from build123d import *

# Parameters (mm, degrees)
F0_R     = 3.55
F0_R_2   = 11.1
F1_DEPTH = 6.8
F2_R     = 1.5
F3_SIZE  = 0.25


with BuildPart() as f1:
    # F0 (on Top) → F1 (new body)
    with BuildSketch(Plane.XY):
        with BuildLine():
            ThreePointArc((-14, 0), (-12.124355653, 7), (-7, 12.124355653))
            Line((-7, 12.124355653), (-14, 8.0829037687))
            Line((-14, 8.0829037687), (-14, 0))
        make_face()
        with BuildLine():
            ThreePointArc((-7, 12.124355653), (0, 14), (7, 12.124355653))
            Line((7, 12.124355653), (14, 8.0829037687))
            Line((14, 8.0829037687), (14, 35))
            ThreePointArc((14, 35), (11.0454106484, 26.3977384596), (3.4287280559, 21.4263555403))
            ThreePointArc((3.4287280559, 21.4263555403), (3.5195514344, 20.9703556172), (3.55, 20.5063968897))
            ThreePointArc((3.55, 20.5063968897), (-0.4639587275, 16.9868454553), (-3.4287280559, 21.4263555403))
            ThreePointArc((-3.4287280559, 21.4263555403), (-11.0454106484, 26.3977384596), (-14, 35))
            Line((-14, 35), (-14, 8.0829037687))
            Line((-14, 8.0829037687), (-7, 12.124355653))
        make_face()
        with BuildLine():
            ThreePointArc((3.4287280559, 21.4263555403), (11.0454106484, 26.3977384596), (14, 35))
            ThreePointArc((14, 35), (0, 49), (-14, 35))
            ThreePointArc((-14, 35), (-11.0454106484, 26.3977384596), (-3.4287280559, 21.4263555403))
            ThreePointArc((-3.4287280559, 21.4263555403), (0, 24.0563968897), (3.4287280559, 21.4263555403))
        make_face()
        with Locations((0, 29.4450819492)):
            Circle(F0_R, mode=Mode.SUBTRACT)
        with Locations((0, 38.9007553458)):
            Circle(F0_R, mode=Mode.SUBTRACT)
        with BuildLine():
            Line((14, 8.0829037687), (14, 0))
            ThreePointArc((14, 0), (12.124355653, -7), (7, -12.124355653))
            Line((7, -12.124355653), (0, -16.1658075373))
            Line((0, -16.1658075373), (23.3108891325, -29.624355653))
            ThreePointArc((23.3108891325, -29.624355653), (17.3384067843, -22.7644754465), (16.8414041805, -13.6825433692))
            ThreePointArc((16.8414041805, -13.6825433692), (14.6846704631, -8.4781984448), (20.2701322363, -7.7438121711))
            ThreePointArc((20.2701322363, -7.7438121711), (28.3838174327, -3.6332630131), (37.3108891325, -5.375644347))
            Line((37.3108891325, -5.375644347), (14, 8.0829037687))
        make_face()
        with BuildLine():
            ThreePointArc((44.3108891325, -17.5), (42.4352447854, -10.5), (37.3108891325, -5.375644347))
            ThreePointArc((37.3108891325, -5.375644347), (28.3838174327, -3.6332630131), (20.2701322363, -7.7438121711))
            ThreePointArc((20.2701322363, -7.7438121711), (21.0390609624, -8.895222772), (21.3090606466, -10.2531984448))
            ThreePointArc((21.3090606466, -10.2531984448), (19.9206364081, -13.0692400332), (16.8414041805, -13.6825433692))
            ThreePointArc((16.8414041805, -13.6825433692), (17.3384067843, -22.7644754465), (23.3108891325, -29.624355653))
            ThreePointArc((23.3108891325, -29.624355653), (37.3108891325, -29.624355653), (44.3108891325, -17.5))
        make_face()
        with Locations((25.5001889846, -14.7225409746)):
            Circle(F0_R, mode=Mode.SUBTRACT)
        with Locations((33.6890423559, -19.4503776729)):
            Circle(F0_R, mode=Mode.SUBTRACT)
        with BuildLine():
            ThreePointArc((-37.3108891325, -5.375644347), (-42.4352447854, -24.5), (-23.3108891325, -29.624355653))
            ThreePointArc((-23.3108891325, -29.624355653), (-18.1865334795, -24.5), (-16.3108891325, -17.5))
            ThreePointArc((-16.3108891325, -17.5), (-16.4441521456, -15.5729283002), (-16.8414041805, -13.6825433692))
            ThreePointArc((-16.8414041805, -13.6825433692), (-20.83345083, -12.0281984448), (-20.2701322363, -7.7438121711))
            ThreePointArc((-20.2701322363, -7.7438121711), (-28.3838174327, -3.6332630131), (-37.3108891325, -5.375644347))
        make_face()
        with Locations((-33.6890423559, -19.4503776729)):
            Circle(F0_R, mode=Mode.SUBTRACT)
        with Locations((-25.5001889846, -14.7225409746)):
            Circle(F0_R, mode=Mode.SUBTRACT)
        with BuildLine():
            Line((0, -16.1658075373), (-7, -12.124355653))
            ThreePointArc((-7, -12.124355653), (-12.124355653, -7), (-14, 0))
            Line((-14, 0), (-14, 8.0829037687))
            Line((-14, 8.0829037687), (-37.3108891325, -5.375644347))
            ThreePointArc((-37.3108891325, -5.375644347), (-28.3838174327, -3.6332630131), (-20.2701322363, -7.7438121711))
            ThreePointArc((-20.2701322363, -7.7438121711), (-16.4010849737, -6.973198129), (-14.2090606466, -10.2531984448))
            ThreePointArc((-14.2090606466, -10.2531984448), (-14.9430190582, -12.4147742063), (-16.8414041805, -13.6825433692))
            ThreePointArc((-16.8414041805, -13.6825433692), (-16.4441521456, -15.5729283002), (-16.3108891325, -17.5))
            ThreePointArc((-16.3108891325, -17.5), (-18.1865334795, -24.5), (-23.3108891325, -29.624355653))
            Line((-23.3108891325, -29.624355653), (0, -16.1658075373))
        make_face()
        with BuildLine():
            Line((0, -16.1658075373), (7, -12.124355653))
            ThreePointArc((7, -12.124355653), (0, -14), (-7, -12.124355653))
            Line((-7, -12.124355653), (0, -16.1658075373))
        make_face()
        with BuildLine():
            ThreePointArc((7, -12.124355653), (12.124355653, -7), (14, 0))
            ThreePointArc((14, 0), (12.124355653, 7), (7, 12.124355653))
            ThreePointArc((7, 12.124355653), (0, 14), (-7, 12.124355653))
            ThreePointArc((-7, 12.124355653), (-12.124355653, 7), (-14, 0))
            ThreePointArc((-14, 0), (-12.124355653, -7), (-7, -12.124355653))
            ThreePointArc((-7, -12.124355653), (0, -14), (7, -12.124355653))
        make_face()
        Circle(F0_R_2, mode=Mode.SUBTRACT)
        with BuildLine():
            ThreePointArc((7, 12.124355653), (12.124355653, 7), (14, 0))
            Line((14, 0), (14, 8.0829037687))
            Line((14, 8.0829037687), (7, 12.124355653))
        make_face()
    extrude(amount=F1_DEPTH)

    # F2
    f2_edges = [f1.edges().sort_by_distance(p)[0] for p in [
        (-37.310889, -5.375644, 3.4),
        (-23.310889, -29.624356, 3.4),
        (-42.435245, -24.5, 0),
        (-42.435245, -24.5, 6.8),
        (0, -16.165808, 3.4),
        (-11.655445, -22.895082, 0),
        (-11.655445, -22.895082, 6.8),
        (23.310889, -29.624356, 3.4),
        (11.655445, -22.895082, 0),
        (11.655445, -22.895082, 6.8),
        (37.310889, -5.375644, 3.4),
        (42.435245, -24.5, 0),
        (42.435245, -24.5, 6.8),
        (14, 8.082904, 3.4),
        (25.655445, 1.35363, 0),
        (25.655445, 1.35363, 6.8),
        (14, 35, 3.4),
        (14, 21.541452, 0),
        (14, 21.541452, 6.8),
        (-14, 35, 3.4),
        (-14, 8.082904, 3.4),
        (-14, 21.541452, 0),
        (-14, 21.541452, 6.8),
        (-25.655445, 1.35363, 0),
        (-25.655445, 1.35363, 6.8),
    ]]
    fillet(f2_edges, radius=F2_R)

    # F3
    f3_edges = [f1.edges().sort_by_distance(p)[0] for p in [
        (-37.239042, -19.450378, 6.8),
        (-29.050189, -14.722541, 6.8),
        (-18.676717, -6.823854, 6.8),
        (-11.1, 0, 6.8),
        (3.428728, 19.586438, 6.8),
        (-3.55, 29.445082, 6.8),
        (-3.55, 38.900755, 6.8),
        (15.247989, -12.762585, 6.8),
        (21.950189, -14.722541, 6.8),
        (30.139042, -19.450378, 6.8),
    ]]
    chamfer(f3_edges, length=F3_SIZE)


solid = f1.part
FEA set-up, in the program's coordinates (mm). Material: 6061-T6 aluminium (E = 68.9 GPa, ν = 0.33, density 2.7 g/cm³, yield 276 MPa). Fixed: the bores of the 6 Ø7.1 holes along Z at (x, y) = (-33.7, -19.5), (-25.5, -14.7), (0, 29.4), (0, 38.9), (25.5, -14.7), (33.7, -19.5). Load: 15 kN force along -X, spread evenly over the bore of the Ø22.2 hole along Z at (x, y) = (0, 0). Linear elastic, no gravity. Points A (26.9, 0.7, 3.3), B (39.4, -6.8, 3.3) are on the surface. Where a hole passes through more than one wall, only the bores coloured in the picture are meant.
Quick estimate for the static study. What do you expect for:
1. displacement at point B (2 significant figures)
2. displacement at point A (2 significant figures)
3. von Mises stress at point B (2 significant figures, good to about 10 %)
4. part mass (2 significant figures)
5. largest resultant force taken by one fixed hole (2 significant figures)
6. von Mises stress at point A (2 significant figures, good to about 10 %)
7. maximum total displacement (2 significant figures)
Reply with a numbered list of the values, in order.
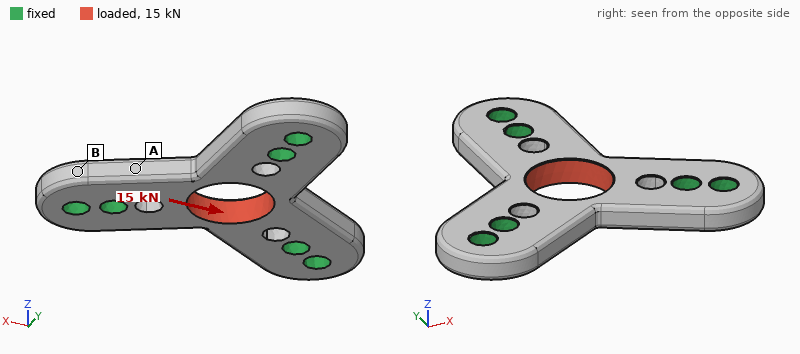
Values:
1. 8.1 µm
2. 21 µm
3. 19 MPa
4. 50 g
5. 5.4 kN
6. 56 MPa
7. 44 µm
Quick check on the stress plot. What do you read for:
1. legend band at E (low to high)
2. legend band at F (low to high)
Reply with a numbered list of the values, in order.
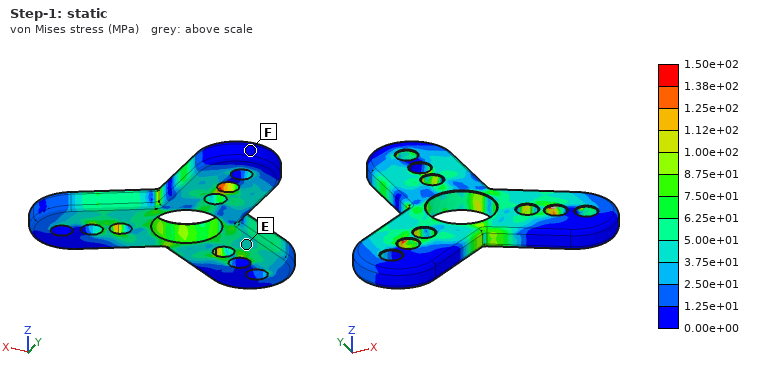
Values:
1. 3.75e+01 to 5.00e+01 MPa
2. 0.00e+00 to 1.25e+01 MPa
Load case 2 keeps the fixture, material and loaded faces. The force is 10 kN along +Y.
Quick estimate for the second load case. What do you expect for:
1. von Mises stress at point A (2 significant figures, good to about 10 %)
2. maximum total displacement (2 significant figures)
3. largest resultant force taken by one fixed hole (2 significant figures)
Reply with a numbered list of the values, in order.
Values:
1. 20 MPa
2. 33 µm
3. 3.5 kN
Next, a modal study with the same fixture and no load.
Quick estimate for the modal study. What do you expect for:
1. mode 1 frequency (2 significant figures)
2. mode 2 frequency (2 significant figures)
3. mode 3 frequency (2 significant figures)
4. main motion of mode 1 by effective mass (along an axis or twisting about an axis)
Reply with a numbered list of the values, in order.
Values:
1. 13 kHz
2. 17 kHz
3. 17 kHz
4. along Z
